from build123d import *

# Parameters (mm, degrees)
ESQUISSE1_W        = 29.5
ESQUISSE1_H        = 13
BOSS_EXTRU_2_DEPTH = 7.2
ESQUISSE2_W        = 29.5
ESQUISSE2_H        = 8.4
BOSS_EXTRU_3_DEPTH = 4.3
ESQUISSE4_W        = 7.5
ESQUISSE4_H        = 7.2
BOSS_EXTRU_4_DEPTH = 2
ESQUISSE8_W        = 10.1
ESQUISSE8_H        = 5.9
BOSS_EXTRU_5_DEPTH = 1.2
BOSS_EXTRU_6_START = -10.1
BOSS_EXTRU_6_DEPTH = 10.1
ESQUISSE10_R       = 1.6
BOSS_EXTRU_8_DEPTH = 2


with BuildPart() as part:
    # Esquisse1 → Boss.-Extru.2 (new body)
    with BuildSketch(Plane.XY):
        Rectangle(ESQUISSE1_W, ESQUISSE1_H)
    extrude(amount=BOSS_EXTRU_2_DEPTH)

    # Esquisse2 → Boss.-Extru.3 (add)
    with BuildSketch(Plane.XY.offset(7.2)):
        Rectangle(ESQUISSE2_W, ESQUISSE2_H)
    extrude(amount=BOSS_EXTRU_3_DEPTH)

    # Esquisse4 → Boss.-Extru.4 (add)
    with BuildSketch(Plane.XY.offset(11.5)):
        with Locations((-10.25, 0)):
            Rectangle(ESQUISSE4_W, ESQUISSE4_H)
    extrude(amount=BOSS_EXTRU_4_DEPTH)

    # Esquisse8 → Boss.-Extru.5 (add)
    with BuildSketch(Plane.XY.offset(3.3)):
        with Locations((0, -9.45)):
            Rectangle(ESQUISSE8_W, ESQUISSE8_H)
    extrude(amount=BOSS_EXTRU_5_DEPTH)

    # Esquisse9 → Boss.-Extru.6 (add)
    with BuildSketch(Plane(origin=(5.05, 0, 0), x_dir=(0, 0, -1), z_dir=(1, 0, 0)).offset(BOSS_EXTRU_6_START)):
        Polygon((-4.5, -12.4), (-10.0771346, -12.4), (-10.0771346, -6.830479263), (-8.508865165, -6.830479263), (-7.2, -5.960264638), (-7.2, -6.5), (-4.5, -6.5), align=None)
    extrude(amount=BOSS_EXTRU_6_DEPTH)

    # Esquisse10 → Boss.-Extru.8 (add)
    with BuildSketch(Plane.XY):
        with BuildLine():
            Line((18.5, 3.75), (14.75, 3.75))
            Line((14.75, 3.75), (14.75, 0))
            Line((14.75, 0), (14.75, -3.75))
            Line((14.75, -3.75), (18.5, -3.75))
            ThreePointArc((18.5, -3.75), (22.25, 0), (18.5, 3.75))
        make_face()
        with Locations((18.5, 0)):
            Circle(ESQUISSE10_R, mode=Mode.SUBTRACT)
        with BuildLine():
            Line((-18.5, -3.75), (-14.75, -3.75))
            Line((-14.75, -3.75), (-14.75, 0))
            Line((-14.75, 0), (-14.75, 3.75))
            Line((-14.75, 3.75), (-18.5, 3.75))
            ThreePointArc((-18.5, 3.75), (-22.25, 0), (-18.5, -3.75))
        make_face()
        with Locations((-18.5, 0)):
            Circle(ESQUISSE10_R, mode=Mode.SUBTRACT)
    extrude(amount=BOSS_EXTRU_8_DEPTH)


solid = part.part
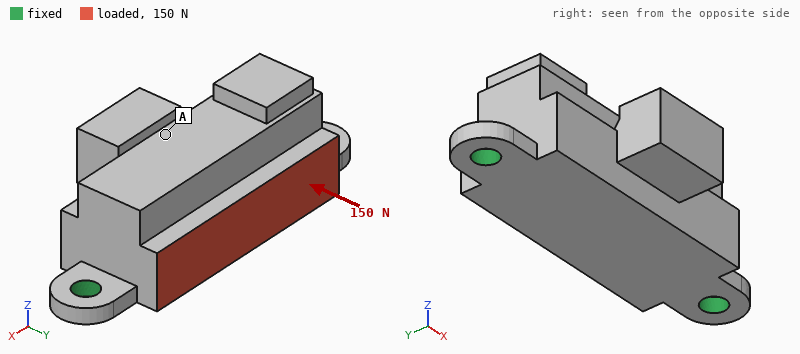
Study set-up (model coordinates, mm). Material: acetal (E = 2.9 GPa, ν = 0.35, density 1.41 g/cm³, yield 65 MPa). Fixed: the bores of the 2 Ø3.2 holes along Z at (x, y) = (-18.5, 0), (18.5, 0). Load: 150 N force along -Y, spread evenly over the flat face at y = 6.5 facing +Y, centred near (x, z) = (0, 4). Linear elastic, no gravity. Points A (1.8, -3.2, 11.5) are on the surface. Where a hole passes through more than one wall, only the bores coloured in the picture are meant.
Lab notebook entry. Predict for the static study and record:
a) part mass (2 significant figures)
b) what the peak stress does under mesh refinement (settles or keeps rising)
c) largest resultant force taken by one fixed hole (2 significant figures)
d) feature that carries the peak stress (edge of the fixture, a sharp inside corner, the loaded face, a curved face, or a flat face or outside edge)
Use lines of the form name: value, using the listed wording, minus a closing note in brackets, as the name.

part mass: 6.3 g
what the peak stress does under mesh refinement: keeps rising
largest resultant force taken by one fixed hole: 75 N
feature that carries the peak stress: edge of the fixture
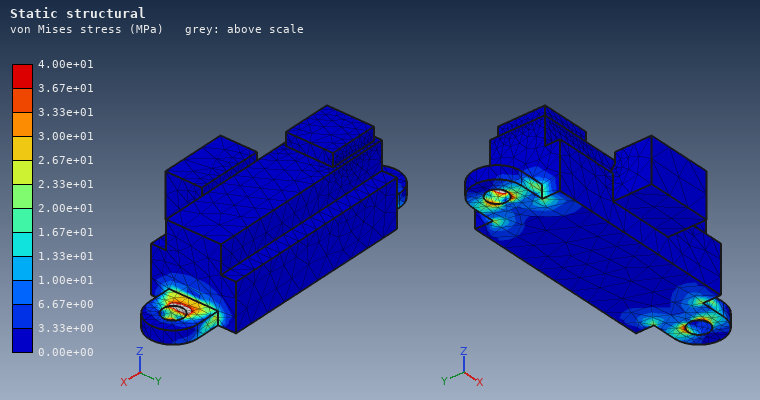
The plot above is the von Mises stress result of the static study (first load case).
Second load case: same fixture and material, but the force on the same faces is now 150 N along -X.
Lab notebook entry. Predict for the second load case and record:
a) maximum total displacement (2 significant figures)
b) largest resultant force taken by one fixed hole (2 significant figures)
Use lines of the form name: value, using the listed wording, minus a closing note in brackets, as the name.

maximum total displacement: 25 µm
largest resultant force taken by one fixed hole: 81 N
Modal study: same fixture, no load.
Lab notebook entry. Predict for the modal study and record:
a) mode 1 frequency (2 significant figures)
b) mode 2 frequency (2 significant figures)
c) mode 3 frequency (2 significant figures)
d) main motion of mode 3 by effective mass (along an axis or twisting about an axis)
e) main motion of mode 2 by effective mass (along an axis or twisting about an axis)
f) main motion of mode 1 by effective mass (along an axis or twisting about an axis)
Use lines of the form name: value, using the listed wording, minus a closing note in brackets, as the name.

mode 1 frequency: 1200 Hz
mode 2 frequency: 3400 Hz
mode 3 frequency: 5200 Hz
main motion of mode 3 by effective mass: along Y
main motion of mode 2 by effective mass: along Z
main motion of mode 1 by effective mass: along Y
